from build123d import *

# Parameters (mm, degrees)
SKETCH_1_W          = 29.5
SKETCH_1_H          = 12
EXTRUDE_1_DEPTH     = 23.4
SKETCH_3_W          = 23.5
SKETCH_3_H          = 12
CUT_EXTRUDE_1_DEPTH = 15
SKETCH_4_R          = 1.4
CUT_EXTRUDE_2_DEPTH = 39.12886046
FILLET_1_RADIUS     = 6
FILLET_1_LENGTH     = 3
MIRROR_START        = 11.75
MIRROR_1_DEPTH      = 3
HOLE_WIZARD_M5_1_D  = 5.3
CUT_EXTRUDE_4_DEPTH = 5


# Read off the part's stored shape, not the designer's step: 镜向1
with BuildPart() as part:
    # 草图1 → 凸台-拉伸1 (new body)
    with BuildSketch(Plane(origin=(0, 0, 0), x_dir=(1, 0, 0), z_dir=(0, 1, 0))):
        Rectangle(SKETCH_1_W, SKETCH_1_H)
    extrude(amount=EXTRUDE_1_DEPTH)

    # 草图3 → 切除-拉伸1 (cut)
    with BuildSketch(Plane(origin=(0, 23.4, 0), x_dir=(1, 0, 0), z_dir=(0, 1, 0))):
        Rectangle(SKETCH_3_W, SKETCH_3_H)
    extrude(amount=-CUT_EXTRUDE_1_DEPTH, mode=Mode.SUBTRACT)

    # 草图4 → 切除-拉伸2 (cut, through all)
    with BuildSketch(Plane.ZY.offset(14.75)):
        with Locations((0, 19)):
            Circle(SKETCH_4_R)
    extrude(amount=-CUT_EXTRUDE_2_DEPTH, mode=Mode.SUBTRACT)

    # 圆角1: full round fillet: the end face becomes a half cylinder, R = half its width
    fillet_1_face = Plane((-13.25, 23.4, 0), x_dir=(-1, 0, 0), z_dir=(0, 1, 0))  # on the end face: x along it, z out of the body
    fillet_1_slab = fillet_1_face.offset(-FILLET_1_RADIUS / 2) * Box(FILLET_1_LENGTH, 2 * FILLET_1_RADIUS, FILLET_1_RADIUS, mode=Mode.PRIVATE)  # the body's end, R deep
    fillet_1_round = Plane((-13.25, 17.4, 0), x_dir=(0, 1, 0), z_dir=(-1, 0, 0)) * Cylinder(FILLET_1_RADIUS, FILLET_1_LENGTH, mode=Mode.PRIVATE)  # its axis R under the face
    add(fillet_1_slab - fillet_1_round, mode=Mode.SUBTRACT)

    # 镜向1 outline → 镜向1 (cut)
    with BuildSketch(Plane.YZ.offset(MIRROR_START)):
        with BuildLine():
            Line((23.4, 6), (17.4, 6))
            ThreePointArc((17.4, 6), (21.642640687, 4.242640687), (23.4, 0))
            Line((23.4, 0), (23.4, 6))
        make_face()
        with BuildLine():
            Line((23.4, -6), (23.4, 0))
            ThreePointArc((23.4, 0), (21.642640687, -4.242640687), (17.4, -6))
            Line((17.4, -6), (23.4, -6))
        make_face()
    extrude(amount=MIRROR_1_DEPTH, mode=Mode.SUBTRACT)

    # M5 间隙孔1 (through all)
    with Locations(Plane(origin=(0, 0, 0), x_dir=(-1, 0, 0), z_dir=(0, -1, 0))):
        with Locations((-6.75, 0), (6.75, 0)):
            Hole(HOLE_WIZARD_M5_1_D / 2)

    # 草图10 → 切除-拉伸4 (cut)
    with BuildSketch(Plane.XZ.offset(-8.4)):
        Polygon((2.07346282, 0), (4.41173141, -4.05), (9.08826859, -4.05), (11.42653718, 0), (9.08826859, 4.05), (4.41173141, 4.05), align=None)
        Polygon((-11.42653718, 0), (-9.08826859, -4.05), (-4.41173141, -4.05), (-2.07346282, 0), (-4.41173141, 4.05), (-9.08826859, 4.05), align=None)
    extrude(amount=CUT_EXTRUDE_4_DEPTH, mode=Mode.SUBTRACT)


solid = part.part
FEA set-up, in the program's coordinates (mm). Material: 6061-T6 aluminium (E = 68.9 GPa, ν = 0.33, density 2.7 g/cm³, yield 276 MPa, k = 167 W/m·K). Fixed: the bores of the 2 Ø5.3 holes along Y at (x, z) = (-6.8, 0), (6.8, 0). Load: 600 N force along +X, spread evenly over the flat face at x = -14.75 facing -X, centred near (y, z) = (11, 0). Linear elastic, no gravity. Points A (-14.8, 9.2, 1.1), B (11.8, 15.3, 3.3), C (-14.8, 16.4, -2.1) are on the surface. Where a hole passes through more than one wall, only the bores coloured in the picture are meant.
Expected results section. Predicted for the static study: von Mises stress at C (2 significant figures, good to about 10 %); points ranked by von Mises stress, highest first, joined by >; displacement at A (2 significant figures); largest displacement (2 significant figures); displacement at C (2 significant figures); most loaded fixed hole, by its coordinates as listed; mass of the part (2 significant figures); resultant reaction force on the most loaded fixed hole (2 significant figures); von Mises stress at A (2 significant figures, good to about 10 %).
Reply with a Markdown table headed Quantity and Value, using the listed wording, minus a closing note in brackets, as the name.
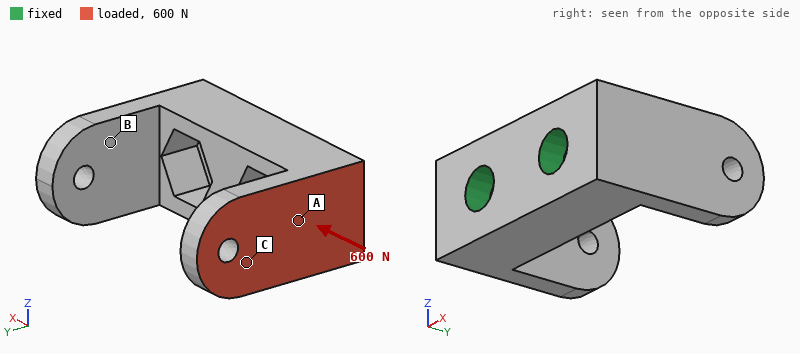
| Quantity | Value |
|---|---|
| von Mises stress at C | 31 MPa |
| points ranked by von Mises stress, highest first, joined by > | A > C > B |
| displacement at A | 0.025 mm |
| largest displacement | 0.15 mm |
| displacement at C | 0.082 mm |
| most loaded fixed hole, by its coordinates as listed | (6.8, 0) |
| mass of the part | 8.7 g |
| resultant reaction force on the most loaded fixed hole | 430 N |
| von Mises stress at A | 110 MPa |
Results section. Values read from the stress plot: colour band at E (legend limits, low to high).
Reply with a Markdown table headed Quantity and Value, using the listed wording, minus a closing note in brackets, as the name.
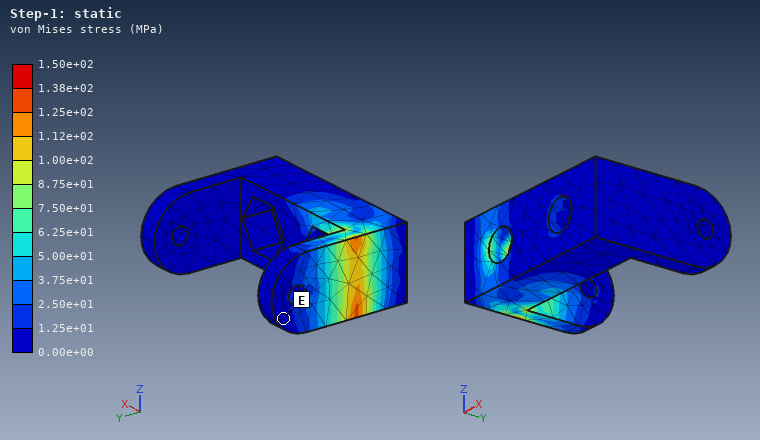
| Quantity | Value |
|---|---|
| colour band at E | 0.00e+00 to 1.25e+01 MPa |
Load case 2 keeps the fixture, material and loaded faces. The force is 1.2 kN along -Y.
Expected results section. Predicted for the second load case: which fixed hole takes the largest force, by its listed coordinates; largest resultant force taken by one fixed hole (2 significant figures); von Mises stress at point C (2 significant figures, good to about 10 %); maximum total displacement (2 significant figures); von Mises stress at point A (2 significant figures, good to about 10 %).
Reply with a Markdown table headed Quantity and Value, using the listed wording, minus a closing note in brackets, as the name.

| Quantity | Value |
|---|---|
| which fixed hole takes the largest force, by its listed coordinates | (-6.8, 0) |
| largest resultant force taken by one fixed hole | 1.6 kN |
| von Mises stress at point C | 39 MPa |
| maximum total displacement | 0.12 mm |
| von Mises stress at point A | 75 MPa |
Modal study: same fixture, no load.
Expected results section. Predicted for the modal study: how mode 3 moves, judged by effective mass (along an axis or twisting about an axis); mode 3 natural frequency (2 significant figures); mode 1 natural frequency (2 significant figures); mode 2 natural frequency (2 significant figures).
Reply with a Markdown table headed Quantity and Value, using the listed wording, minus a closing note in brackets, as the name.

| Quantity | Value |
|---|---|
| how mode 3 moves, judged by effective mass | along Z |
| mode 3 natural frequency | 13 kHz |
| mode 1 natural frequency | 8900 Hz |
| mode 2 natural frequency | 9000 Hz |
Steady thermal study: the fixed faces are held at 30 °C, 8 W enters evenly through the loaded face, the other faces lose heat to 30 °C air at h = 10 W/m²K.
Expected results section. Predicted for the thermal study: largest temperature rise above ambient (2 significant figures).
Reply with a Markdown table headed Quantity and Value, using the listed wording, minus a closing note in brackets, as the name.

| Quantity | Value |
|---|---|
| largest temperature rise above ambient | 13 K |
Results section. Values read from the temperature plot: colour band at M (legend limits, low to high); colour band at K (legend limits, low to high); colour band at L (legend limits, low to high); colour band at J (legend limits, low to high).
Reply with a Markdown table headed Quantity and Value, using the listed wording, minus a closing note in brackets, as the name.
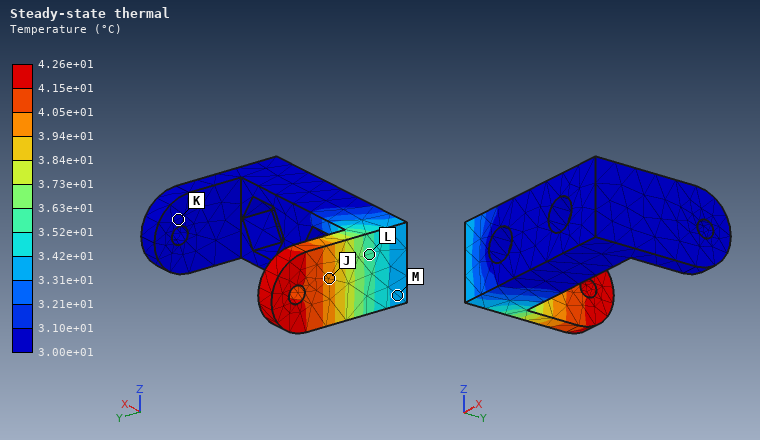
| Quantity | Value |
|---|---|
| colour band at M | 3.31e+01 to 3.42e+01 °C |
| colour band at K | 3.00e+01 to 3.10e+01 °C |
| colour band at L | 3.52e+01 to 3.63e+01 °C |
| colour band at J | 3.94e+01 to 4.05e+01 °C |
